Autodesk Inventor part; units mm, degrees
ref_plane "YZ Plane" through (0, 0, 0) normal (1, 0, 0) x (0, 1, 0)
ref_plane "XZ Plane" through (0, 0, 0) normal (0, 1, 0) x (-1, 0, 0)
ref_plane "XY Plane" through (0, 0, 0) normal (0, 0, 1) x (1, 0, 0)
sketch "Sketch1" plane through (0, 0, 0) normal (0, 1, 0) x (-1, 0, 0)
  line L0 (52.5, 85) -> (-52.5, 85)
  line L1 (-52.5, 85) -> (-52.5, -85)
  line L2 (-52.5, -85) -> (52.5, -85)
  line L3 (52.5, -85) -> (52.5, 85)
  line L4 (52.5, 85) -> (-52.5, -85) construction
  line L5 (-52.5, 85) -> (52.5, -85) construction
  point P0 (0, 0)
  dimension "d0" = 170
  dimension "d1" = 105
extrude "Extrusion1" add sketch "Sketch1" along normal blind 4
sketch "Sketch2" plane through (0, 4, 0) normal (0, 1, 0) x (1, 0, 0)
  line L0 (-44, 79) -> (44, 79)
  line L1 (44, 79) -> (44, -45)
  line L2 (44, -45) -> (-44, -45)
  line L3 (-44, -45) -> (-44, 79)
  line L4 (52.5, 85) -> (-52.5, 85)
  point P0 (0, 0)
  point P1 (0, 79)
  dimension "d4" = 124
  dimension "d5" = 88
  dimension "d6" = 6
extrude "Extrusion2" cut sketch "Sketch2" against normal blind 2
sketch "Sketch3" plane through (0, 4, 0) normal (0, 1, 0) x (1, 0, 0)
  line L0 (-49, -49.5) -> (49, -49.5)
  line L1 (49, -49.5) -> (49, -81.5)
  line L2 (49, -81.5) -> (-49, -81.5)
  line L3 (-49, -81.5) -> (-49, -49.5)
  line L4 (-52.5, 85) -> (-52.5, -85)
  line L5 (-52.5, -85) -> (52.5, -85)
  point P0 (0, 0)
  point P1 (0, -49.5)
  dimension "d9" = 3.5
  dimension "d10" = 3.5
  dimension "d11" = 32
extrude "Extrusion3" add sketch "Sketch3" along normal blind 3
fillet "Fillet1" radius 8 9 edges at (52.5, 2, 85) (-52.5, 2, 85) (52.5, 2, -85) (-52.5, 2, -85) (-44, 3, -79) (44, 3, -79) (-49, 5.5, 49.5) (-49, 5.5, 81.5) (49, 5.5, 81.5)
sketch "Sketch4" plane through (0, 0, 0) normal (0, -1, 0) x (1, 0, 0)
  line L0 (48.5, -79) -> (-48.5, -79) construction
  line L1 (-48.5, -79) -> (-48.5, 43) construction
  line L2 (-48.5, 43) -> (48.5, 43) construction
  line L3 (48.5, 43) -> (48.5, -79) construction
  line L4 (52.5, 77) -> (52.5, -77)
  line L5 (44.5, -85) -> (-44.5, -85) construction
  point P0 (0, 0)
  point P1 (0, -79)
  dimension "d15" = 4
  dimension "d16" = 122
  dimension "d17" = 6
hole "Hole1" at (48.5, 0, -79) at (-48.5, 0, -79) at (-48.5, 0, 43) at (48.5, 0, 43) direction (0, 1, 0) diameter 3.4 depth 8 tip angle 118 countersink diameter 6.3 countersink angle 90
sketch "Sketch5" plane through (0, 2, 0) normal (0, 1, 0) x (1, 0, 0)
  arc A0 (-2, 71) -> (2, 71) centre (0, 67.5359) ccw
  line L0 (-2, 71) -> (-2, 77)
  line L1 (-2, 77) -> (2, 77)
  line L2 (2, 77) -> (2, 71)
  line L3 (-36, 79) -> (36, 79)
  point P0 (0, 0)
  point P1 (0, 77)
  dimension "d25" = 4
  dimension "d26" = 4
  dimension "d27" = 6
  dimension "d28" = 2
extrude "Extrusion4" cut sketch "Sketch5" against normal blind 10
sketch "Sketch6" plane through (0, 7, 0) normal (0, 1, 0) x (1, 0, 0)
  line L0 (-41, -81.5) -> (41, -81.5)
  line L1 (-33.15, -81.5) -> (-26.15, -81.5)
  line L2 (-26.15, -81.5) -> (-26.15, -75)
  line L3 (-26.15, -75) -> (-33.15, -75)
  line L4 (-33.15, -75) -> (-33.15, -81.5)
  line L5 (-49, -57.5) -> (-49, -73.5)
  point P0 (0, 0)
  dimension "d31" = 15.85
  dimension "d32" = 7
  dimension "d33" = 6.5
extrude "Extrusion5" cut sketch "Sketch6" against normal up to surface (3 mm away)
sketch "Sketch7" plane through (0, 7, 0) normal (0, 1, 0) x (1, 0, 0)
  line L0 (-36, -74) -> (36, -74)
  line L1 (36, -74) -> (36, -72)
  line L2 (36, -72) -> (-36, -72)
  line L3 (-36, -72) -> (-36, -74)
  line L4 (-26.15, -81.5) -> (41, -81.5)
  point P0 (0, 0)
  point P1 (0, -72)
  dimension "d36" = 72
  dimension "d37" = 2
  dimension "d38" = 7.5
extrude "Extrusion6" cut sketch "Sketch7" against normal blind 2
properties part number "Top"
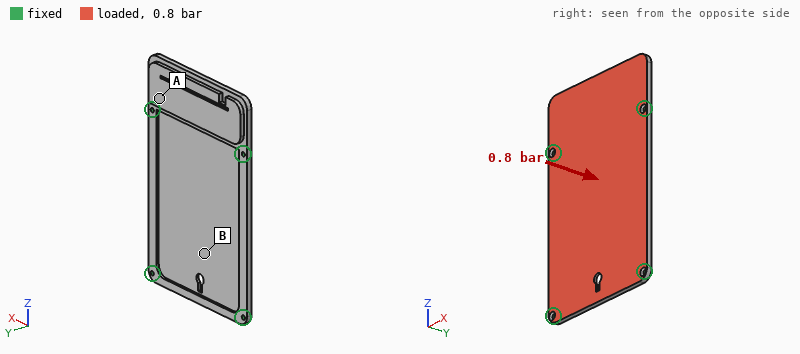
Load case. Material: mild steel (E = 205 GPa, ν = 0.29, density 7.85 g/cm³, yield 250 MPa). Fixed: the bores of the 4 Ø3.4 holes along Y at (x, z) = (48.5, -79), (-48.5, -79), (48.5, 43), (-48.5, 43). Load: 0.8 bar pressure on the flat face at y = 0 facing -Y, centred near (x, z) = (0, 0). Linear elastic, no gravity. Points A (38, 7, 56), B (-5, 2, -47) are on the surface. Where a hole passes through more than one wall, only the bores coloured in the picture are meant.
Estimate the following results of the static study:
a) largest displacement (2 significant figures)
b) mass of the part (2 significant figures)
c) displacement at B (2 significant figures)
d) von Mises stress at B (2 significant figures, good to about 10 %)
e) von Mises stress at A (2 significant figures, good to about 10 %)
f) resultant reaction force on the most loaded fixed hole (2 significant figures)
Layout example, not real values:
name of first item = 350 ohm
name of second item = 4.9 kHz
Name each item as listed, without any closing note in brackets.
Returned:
largest displacement = 0.26 mm
mass of the part = 450 g
displacement at B = 0.20 mm
von Mises stress at B = 33 MPa
von Mises stress at A = 14 MPa
resultant reaction force on the most loaded fixed hole = 740 N
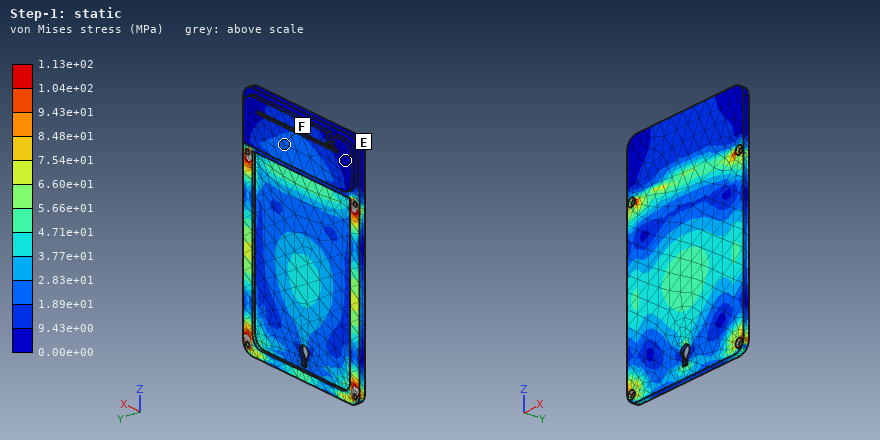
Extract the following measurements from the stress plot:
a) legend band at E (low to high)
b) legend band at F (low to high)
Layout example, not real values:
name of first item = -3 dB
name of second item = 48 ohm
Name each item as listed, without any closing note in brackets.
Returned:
legend band at E = 0.00e+00 to 9.43e+00 MPa
legend band at F = 1.89e+01 to 2.83e+01 MPa
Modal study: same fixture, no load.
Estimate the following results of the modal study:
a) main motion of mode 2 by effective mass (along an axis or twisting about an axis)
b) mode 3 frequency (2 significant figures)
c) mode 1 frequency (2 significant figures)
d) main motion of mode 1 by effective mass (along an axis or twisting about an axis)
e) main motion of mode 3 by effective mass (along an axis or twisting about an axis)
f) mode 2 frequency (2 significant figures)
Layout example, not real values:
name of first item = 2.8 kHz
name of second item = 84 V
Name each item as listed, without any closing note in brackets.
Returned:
main motion of mode 2 by effective mass = along Y
mode 3 frequency = 1300 Hz
mode 1 frequency = 780 Hz
main motion of mode 1 by effective mass = twisting about X
main motion of mode 3 by effective mass = twisting about Z
mode 2 frequency = 930 Hz
